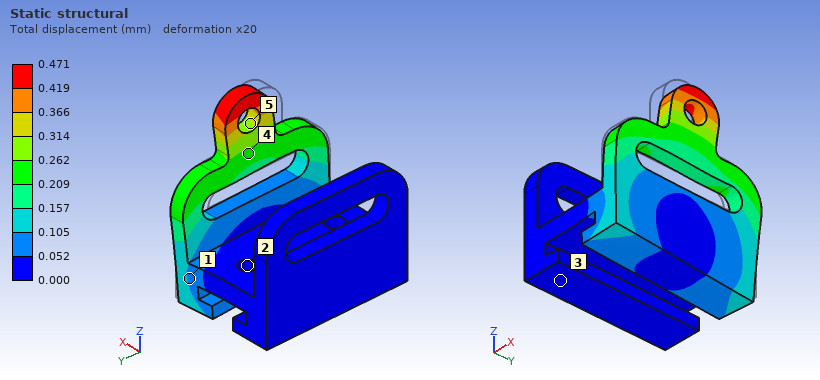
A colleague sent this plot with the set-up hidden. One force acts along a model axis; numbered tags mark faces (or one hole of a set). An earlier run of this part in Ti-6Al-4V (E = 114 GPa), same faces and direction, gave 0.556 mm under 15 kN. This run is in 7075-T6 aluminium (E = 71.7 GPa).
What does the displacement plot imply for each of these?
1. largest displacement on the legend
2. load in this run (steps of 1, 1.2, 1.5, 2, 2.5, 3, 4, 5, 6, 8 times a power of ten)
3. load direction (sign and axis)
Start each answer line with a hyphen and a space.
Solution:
- 0.471 mm
- 8 kN
- +Y
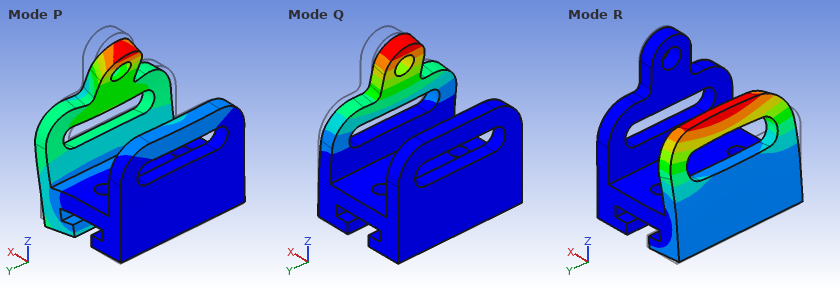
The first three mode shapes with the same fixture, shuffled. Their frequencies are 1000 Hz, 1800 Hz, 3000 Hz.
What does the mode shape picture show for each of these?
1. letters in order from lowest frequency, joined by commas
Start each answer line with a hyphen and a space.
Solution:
- Q, R, P
